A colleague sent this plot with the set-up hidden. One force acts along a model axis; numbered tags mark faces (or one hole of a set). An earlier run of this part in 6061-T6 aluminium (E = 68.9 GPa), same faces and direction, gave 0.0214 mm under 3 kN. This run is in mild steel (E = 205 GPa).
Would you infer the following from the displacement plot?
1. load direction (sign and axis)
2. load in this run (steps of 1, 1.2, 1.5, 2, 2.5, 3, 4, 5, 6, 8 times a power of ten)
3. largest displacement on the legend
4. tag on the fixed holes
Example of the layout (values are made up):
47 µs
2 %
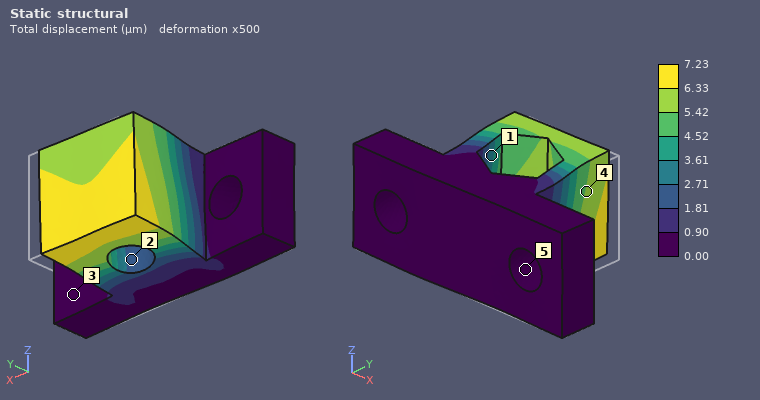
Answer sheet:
-X
3 kN
7.23 µm
5
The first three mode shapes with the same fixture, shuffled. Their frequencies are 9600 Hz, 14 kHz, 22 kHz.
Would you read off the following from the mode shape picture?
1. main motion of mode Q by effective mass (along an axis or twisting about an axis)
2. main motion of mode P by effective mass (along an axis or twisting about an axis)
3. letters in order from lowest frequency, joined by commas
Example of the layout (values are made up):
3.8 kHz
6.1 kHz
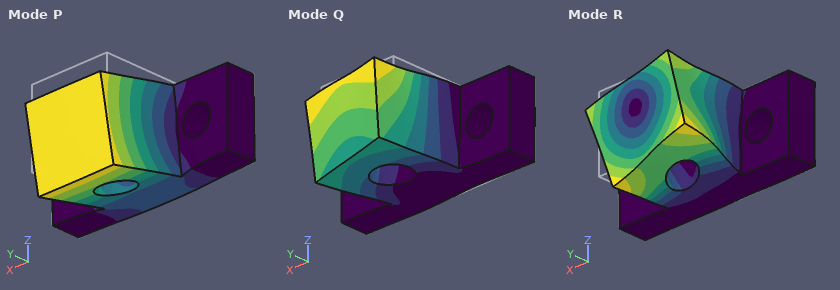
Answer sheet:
along X
along Z
P, Q, R
